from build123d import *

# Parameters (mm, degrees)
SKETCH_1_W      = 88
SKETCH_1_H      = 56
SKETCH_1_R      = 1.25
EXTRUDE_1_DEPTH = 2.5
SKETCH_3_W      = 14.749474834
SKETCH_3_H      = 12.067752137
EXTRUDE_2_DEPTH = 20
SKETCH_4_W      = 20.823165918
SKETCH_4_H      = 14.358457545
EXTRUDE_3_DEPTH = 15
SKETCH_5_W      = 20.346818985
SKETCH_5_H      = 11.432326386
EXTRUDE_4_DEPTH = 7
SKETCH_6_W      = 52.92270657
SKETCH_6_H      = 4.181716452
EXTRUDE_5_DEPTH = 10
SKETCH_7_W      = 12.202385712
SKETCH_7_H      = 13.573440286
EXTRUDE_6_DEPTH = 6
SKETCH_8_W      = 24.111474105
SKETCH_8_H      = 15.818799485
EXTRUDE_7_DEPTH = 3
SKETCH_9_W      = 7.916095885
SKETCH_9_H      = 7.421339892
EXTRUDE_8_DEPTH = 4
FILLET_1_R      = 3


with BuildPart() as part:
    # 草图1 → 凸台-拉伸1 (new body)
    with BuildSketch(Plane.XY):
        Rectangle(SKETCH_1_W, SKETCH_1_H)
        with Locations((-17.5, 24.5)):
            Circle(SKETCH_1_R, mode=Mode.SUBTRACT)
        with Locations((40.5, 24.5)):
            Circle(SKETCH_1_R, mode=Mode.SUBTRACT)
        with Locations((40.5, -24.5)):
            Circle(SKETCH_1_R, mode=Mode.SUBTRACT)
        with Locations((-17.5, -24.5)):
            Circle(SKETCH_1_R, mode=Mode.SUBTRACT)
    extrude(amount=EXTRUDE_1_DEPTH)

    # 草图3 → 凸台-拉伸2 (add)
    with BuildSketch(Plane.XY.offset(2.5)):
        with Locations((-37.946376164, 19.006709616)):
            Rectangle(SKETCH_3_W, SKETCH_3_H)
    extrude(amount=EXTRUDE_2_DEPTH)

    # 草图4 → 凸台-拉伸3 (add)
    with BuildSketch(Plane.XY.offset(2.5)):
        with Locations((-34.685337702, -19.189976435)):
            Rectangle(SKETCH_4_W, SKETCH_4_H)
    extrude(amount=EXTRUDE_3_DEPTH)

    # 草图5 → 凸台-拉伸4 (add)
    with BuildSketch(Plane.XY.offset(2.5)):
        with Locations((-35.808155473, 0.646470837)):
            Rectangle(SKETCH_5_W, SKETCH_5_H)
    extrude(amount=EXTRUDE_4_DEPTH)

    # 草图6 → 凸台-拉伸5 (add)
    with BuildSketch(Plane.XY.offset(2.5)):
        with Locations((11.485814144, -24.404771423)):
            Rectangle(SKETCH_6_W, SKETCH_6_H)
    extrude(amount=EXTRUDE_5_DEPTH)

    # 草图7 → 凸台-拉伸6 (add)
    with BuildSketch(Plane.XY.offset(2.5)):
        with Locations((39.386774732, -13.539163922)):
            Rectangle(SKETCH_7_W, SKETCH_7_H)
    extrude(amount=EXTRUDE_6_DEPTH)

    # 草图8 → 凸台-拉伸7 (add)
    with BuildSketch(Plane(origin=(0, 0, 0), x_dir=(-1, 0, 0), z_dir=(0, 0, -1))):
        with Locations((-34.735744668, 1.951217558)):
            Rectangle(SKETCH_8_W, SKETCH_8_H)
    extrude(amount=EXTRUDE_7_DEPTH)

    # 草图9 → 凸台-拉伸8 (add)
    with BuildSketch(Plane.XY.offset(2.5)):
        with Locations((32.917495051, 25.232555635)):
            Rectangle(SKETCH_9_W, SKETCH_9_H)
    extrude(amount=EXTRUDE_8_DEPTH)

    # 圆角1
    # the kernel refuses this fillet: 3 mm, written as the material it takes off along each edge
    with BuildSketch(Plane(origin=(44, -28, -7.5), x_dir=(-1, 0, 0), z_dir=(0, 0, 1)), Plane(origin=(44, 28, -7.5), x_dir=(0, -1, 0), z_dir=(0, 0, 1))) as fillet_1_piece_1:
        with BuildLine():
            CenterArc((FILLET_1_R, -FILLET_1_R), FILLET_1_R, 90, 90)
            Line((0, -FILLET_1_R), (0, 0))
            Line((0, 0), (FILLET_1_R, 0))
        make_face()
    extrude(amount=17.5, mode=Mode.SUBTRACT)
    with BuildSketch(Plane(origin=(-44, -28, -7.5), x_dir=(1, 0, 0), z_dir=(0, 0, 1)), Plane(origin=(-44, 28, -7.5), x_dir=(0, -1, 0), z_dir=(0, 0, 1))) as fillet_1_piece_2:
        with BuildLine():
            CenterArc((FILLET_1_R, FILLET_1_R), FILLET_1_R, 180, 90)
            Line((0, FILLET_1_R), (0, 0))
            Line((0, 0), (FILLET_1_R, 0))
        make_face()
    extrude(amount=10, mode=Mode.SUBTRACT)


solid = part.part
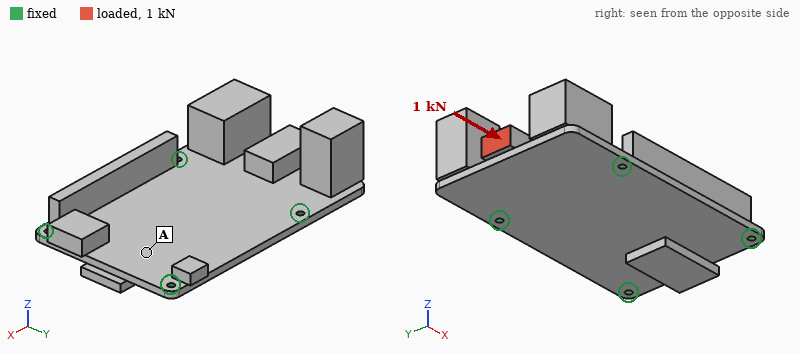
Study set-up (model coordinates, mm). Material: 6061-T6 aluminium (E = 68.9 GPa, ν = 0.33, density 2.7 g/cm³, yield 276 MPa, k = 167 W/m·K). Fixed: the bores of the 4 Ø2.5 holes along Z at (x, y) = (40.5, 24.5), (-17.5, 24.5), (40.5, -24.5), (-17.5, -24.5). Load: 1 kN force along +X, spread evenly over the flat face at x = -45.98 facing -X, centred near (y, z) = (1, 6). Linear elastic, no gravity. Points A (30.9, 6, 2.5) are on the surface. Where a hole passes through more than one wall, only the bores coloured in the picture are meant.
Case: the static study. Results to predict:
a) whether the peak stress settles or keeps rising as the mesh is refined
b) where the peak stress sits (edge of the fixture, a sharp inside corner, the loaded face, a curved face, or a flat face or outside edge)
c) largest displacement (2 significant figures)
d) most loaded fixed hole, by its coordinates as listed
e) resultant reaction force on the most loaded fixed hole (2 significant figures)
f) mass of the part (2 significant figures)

keeps rising
edge of the fixture
0.39 mm
(-17.5, 24.5)
400 N
72 g
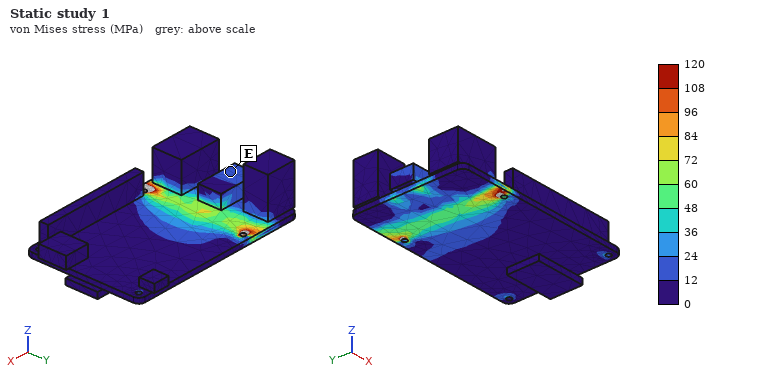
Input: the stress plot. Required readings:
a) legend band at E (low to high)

12 to 24 MPa
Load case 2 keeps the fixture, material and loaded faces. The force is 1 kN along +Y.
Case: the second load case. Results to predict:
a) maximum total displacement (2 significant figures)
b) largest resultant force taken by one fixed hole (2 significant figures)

64 µm
750 N
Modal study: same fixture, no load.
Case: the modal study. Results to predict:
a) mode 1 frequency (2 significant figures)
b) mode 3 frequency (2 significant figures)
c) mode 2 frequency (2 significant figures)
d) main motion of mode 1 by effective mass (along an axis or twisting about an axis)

920 Hz
2800 Hz
2200 Hz
along Z
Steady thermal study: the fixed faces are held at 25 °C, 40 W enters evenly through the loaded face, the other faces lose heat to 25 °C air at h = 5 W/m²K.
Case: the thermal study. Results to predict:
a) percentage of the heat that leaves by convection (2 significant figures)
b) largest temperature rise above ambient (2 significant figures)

3.2 %
74 K
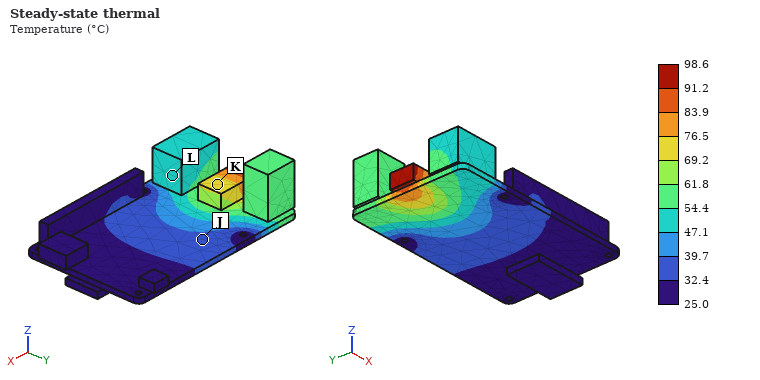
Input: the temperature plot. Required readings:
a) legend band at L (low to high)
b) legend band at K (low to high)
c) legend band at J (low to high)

47.1 to 54.4 °C
69.2 to 76.5 °C
32.4 to 39.7 °C
